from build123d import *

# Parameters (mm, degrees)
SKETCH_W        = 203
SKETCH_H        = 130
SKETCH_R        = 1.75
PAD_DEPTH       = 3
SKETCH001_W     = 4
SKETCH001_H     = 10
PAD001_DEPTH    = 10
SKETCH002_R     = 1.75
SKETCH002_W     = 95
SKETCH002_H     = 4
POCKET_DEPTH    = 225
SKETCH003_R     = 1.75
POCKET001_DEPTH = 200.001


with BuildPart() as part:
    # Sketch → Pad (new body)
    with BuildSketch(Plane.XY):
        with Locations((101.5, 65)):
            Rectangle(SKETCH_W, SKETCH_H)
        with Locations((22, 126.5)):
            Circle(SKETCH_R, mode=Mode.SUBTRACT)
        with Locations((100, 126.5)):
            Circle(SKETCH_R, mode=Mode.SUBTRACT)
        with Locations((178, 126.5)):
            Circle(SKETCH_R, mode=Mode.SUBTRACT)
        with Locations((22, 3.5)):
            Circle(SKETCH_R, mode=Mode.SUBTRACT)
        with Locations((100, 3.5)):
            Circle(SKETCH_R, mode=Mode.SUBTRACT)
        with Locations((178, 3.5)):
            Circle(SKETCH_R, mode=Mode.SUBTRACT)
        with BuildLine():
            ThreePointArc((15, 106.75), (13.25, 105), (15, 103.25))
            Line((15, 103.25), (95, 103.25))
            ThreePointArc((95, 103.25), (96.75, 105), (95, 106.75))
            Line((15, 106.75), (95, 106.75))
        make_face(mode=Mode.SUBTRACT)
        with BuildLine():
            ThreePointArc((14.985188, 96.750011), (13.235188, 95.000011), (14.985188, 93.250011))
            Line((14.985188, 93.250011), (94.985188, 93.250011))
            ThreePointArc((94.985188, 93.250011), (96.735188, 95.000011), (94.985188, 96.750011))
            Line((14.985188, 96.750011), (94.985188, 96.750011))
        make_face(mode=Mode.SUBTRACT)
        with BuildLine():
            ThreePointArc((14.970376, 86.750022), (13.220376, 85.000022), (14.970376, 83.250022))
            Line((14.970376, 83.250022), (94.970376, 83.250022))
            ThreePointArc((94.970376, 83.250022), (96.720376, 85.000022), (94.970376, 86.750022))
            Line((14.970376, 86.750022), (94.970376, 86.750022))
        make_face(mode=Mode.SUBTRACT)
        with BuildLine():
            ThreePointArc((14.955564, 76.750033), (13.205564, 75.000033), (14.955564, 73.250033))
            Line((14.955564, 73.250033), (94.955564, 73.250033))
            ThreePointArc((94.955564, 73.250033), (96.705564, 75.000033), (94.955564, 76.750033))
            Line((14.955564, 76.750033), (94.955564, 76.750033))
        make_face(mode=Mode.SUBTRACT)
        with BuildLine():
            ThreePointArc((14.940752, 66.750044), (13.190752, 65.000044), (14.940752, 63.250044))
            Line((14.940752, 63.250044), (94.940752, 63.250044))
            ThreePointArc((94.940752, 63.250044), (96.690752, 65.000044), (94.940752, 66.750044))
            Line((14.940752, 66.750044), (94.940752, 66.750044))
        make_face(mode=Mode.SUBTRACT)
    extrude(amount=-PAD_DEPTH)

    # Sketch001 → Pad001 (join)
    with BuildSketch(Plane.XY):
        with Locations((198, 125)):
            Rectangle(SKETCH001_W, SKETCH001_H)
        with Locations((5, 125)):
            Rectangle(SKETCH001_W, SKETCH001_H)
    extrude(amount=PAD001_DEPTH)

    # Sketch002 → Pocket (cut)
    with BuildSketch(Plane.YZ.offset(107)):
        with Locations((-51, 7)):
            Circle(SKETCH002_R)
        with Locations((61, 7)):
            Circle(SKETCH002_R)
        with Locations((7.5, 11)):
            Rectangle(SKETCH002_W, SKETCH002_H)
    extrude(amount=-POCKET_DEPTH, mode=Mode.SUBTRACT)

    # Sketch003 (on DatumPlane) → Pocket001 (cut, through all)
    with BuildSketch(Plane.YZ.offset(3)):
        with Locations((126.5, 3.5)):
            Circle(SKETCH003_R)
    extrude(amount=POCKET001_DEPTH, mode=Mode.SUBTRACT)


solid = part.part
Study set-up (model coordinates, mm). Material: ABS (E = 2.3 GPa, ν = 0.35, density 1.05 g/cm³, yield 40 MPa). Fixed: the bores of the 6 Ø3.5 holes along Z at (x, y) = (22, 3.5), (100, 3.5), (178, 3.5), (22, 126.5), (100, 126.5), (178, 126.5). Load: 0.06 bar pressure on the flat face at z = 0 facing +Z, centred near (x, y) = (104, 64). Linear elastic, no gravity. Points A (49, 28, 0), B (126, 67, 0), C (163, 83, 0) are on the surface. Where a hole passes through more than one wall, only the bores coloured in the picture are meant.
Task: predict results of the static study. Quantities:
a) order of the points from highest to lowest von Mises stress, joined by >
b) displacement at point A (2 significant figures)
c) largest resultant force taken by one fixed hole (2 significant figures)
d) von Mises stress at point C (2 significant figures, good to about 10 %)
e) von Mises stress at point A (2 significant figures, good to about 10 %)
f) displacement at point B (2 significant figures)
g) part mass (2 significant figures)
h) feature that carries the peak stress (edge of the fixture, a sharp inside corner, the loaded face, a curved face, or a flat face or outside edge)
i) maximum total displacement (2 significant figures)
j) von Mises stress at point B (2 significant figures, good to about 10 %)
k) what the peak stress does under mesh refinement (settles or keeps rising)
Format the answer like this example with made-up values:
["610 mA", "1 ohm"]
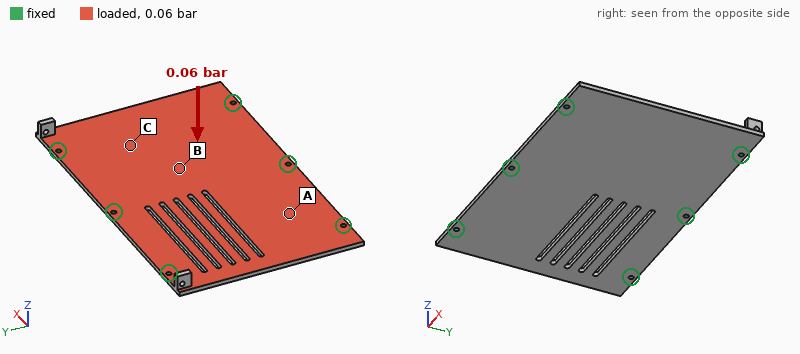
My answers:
["B > C > A", "0.82 mm", "30 N", "2.6 MPa", "1.2 MPa", "1.3 mm", "79 g", "edge of the fixture", "2.2 mm", "3.7 MPa", "keeps rising"]
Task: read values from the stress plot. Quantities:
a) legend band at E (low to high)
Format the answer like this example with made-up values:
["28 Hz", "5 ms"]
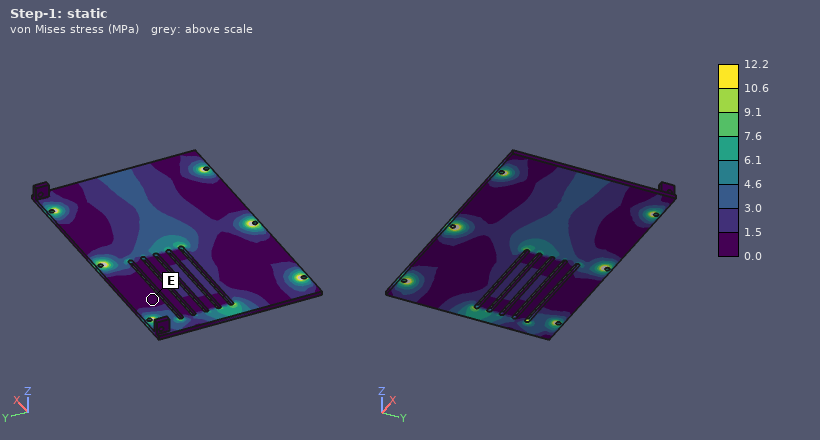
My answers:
["0.0 to 1.5 MPa"]
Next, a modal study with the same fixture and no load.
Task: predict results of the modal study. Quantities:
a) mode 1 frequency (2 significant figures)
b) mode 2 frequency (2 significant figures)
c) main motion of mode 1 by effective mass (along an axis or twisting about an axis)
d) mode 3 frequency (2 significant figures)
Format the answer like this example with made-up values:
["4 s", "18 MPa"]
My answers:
["190 Hz", "250 Hz", "along Z", "330 Hz"]
